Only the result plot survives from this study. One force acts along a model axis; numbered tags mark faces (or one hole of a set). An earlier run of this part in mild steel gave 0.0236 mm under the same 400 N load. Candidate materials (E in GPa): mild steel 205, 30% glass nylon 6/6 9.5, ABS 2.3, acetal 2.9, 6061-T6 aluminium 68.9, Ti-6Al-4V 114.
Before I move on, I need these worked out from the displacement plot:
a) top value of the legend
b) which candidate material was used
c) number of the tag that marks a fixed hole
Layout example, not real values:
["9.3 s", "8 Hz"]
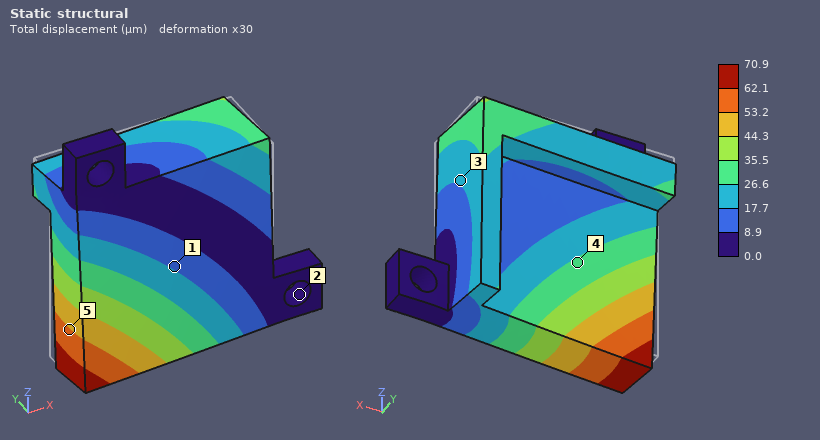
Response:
["70.9 µm", "6061-T6 aluminium", "2"]
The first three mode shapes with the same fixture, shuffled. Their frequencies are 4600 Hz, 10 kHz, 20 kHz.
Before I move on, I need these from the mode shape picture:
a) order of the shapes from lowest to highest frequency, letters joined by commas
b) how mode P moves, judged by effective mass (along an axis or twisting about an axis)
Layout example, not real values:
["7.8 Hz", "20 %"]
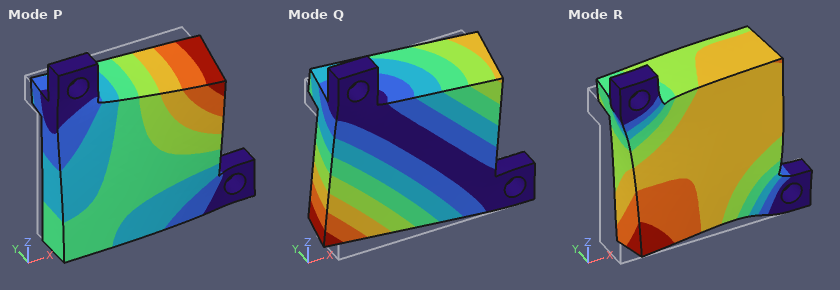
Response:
["Q, P, R", "along Y"]
